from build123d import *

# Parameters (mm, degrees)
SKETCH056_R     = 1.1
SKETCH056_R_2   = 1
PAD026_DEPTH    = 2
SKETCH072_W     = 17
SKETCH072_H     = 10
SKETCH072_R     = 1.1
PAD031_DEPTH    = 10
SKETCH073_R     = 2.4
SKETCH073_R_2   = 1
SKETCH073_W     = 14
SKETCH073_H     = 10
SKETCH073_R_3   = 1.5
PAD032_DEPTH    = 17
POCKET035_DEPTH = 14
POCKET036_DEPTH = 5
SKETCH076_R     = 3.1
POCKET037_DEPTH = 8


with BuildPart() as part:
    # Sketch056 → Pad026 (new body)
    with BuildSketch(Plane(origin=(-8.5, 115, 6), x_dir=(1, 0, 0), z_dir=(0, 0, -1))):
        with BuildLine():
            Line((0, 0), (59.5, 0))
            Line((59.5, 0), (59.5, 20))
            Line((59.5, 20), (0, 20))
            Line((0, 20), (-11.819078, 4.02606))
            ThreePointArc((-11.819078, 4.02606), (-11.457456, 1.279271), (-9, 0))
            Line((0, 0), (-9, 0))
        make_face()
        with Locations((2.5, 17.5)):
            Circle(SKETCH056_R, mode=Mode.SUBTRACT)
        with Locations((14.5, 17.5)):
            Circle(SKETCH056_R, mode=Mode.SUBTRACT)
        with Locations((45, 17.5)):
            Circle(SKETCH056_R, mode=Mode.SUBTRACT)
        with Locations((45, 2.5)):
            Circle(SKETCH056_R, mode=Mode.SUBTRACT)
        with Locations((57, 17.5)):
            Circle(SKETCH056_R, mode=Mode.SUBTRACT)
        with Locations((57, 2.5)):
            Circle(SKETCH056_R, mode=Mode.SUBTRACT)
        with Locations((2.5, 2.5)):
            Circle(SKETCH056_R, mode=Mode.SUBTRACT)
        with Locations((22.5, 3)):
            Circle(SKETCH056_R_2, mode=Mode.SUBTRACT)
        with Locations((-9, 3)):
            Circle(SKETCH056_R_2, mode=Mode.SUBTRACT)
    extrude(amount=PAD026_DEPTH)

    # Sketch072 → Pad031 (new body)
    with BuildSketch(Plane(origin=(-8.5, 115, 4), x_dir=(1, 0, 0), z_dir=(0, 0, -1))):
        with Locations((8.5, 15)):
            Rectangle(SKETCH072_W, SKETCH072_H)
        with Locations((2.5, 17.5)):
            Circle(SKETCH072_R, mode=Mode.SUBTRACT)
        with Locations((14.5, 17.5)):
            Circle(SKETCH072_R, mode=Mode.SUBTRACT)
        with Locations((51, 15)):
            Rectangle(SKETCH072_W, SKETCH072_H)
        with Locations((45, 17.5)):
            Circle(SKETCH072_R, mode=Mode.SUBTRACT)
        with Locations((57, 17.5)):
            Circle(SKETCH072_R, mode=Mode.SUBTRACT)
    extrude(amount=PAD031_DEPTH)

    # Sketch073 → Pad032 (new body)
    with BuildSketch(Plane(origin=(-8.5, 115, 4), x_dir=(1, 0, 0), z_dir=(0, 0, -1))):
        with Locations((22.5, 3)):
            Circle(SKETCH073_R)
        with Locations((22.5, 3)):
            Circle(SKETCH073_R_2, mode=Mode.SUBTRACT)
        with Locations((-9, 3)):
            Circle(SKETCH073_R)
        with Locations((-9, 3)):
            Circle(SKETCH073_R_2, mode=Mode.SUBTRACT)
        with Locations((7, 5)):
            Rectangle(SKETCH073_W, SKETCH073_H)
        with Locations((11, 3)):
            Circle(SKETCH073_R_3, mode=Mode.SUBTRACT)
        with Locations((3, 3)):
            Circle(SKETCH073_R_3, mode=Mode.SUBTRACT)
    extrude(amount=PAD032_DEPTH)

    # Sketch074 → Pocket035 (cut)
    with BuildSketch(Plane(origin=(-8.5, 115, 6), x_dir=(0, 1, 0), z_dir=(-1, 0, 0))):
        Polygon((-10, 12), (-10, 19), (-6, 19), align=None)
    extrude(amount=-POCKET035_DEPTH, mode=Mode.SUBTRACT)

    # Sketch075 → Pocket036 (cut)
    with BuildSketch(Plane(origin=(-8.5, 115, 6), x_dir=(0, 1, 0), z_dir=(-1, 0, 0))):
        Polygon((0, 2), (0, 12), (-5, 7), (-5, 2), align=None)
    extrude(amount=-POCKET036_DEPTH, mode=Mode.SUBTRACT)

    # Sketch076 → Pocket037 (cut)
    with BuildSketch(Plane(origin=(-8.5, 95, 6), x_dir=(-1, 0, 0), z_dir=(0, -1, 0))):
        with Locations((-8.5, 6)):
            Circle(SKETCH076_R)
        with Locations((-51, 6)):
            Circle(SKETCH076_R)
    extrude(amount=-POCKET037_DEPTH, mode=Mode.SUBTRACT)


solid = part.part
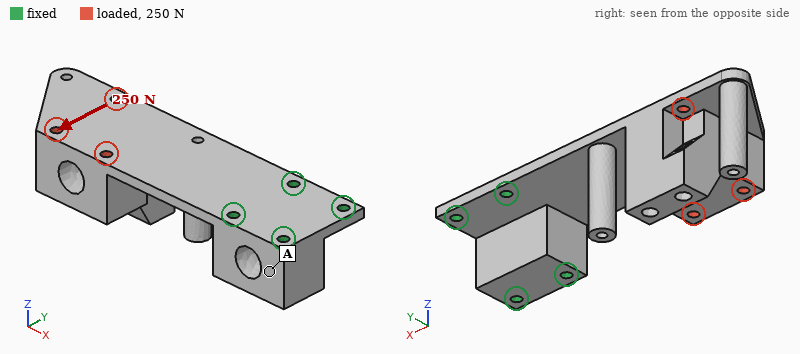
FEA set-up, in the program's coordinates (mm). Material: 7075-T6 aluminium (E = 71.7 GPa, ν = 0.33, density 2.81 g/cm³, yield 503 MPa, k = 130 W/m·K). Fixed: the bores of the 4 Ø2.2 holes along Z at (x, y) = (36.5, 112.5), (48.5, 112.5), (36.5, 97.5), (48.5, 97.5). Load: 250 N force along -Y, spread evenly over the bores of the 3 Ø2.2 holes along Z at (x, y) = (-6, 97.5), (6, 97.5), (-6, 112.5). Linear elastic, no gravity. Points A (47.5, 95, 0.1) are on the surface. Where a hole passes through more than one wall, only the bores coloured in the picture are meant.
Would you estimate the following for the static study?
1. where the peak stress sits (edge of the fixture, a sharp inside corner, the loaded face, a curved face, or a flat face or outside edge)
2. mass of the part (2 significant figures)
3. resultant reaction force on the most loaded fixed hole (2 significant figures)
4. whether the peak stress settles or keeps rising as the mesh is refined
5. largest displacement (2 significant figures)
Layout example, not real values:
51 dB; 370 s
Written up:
edge of the fixture; 22 g; 590 N; keeps rising; 0.41 mm
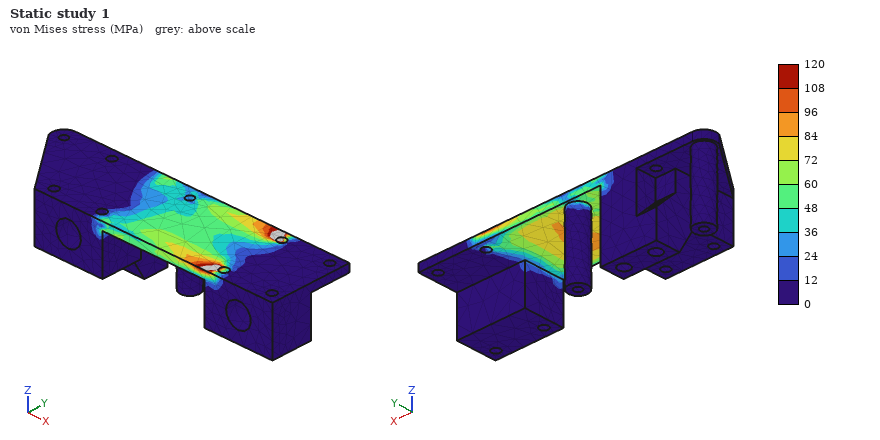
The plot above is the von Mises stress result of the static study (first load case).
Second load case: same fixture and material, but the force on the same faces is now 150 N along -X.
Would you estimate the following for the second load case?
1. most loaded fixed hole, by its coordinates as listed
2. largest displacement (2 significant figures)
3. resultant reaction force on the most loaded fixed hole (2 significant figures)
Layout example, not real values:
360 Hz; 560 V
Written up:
(36.5, 97.5); 0.87 mm; 130 N
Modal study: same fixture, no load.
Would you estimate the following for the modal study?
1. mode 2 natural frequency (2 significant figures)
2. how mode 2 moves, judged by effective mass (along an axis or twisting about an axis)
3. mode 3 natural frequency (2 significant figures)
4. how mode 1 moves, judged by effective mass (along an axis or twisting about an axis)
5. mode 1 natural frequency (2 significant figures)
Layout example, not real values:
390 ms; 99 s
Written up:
1100 Hz; along Y; 2200 Hz; along Z; 310 Hz
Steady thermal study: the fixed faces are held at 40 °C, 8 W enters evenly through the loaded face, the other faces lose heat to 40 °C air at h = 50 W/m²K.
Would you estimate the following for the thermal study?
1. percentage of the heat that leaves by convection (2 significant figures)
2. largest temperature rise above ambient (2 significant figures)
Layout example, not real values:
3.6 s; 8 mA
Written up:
54 %; 27 K
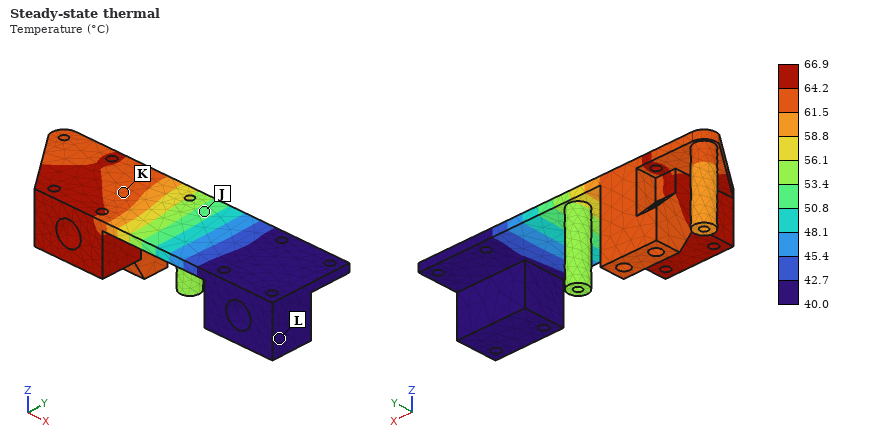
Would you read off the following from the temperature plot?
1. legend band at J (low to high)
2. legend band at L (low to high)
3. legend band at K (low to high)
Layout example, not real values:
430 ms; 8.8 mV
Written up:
50.8 to 53.4 °C; 40.0 to 42.7 °C; 61.5 to 64.2 °C
